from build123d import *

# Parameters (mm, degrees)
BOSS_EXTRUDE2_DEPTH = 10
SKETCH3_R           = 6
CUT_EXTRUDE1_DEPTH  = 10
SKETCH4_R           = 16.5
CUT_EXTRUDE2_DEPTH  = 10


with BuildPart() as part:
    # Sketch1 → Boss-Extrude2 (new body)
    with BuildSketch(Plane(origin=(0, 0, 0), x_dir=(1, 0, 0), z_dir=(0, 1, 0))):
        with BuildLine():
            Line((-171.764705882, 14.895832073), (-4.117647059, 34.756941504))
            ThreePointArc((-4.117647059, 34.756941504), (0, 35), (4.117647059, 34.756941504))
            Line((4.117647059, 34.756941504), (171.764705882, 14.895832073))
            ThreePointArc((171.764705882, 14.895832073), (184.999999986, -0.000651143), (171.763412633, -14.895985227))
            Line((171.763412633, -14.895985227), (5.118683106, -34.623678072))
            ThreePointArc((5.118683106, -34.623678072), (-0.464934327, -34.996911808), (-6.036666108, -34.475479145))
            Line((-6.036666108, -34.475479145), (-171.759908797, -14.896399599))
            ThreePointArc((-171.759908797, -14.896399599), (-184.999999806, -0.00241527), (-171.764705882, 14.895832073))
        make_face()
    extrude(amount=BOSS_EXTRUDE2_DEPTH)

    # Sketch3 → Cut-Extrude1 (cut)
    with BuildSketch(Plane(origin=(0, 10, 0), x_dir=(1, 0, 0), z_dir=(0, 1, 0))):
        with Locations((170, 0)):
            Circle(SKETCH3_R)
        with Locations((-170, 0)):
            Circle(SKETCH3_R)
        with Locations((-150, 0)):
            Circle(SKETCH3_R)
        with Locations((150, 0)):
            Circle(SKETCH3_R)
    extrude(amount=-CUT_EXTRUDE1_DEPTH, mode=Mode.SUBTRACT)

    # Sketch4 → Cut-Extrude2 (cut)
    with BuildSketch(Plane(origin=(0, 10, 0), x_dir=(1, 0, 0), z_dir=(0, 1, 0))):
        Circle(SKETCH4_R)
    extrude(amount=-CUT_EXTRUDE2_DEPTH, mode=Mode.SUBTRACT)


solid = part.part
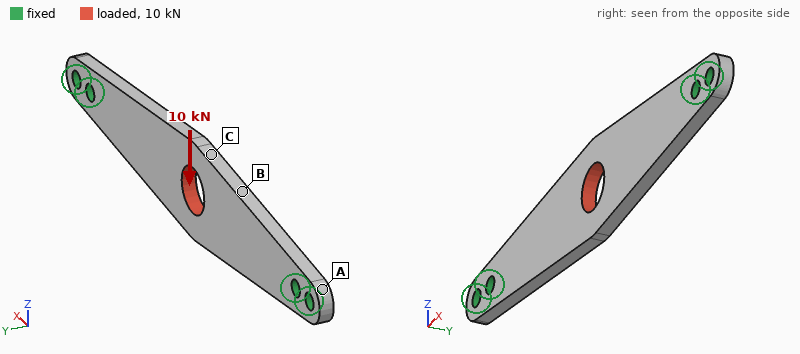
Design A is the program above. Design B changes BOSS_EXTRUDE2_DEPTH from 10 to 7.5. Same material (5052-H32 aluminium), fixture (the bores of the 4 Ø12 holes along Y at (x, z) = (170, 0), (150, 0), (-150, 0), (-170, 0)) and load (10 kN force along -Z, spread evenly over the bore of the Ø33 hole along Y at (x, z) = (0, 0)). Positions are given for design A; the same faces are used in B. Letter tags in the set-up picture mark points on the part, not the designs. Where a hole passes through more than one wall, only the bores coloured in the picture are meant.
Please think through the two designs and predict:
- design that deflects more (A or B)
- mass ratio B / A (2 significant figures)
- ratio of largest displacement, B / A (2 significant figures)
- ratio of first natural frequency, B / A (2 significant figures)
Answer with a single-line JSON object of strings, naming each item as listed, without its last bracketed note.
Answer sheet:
{"design that deflects more": "B", "mass ratio B / A": "0.75", "ratio of largest displacement, B / A": "1.3", "ratio of first natural frequency, B / A": "0.76"}
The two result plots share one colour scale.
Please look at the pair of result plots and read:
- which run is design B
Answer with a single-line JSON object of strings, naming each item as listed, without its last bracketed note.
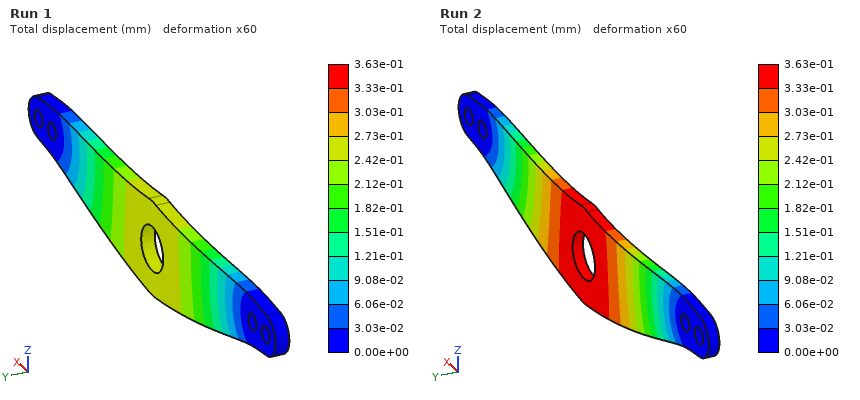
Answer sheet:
{"which run is design B": "Run 2"}
